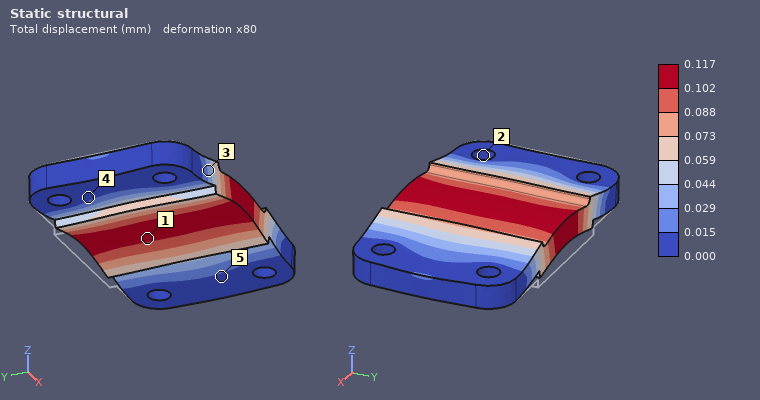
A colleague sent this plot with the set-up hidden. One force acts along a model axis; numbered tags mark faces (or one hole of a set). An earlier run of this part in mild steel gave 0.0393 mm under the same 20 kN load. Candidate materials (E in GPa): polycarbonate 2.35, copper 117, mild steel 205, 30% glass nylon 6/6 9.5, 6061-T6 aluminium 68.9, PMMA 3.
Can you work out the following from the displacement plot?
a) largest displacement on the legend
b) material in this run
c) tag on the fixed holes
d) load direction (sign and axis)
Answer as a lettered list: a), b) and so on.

a) 0.117 mm
b) 6061-T6 aluminium
c) 2
d) +Z
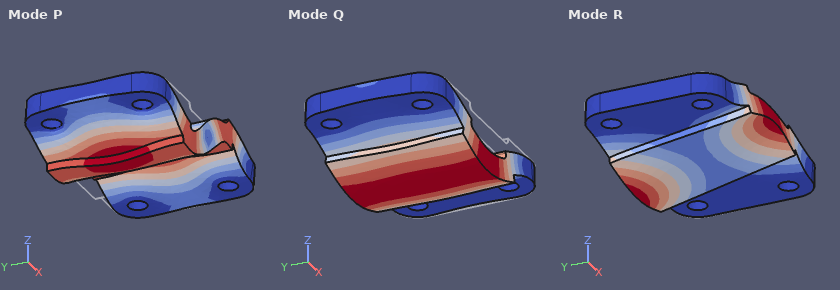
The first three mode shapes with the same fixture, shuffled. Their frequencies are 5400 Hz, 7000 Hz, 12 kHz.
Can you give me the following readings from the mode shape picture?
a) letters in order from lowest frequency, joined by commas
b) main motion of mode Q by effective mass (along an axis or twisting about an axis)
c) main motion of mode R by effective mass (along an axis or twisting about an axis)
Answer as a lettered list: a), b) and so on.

a) Q, R, P
b) along Z
c) twisting about X
